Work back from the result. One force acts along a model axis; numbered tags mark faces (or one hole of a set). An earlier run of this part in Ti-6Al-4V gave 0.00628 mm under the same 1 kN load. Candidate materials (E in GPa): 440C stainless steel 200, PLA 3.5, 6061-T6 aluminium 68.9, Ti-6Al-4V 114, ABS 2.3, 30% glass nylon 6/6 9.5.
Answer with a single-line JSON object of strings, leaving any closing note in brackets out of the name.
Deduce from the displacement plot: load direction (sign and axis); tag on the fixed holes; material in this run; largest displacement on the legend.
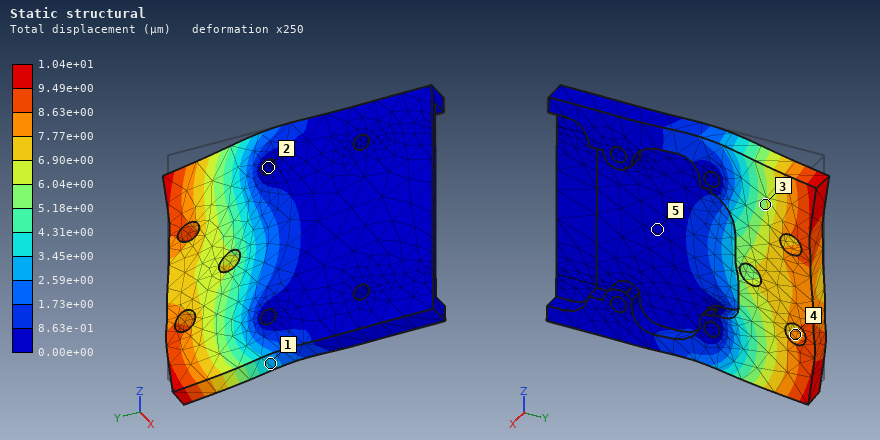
{"load direction": "-Z", "tag on the fixed holes": "2", "material in this run": "6061-T6 aluminium", "largest displacement on the legend": "1.04e+01 µm"}
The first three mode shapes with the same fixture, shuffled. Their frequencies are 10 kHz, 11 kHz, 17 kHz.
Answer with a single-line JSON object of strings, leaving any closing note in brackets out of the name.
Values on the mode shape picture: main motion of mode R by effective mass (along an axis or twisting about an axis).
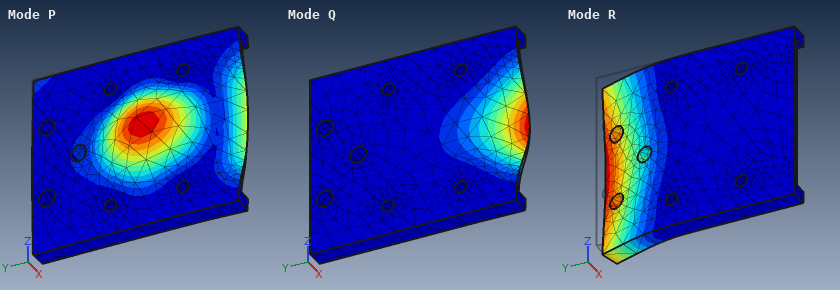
{"main motion of mode R by effective mass": "along X"}
